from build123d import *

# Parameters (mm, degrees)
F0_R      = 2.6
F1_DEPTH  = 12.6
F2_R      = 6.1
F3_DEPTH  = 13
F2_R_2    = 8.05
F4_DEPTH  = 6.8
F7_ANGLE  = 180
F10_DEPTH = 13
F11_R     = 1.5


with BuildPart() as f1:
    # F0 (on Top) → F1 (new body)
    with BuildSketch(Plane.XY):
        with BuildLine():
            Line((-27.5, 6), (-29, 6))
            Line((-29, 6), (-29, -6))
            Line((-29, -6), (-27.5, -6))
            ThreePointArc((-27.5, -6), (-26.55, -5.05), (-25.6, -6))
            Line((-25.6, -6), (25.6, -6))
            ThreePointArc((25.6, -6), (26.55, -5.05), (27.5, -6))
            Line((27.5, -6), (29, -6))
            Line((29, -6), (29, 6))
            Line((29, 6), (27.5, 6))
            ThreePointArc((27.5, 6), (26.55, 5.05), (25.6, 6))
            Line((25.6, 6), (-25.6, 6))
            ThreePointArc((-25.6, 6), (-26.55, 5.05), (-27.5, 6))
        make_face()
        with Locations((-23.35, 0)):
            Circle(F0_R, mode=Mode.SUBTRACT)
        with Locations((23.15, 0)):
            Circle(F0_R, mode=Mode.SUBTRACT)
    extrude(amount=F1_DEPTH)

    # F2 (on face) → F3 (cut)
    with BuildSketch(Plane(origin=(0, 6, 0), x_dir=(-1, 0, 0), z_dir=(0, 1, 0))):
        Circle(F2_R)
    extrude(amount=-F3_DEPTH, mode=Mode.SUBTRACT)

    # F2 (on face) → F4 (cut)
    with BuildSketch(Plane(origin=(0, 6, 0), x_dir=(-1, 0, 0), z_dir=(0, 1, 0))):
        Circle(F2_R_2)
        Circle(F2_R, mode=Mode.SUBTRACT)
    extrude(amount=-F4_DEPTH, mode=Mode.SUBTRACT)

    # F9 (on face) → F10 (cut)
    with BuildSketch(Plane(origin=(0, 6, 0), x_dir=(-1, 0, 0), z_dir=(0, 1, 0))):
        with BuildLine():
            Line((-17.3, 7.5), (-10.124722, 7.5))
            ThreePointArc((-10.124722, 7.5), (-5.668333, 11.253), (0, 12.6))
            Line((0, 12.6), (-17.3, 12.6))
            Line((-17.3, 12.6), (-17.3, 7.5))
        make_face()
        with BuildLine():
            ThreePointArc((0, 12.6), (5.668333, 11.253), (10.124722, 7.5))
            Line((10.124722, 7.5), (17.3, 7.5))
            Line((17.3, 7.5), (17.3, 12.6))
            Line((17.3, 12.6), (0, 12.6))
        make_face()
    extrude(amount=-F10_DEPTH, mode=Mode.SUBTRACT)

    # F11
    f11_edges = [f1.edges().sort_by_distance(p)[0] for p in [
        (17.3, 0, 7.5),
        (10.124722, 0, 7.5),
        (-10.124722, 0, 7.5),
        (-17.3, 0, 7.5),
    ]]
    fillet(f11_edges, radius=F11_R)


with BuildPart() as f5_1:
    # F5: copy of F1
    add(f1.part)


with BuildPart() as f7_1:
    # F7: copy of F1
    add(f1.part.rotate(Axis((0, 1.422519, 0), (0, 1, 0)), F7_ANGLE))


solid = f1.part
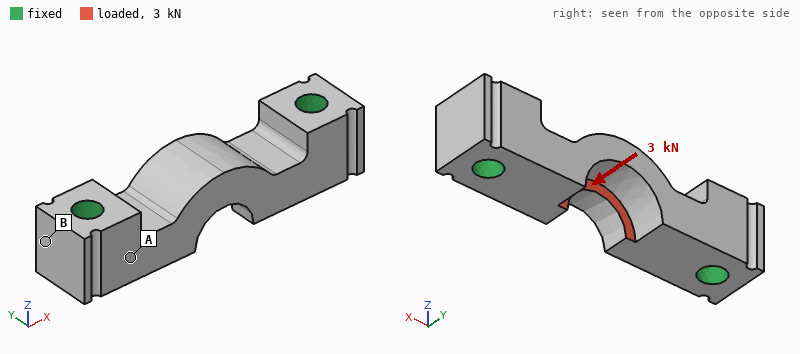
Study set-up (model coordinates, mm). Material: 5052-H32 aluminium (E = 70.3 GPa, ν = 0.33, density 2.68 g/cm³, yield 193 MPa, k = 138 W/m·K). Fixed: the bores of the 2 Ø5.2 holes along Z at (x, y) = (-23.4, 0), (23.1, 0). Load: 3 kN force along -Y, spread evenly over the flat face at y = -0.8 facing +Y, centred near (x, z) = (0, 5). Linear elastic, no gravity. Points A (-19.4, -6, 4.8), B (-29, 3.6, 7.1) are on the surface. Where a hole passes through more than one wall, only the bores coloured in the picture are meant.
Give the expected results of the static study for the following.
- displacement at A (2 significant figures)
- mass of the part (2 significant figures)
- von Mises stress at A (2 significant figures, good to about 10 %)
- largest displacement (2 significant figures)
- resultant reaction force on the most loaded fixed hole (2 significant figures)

7.5 µm
16 g
64 MPa
46 µm
1.5 kN
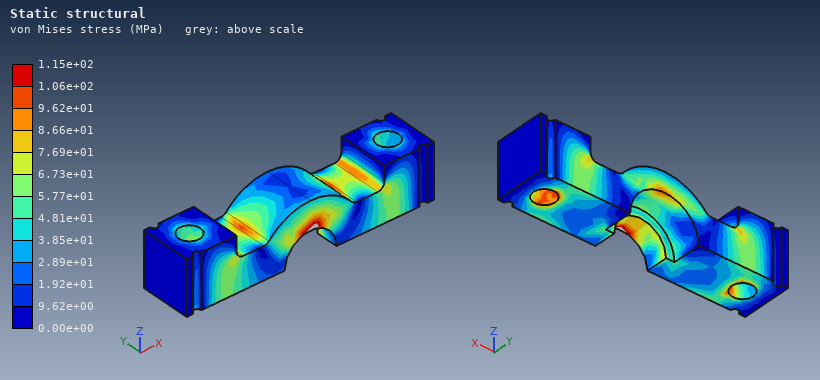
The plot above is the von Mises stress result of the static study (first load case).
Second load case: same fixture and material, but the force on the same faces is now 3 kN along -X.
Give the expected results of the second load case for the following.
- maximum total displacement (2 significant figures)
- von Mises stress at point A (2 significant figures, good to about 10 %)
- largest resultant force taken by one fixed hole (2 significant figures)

9.8 µm
14 MPa
1.5 kN
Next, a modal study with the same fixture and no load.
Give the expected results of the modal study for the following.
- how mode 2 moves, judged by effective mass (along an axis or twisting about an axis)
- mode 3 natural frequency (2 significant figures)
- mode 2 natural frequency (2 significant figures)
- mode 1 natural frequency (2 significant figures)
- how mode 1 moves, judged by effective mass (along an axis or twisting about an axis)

along Z
35 kHz
23 kHz
18 kHz
along Y
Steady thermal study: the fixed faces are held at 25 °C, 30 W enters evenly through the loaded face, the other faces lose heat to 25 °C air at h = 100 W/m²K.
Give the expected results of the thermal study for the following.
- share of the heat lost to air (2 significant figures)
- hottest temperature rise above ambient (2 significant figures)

6.9 %
28 K
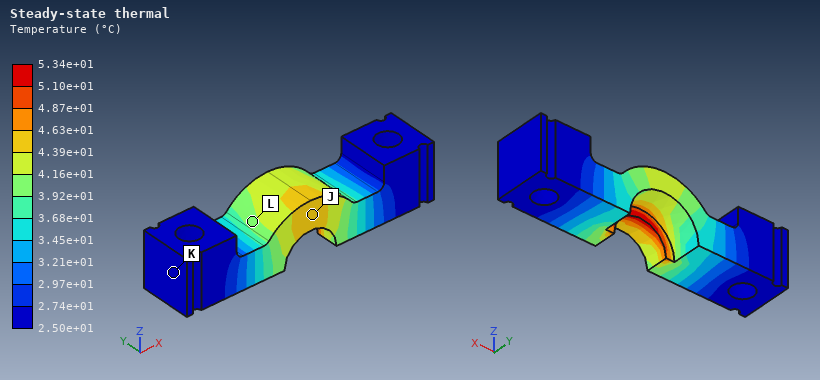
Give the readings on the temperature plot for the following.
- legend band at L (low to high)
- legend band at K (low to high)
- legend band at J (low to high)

3.92e+01 to 4.16e+01 °C
2.50e+01 to 2.74e+01 °C
4.39e+01 to 4.63e+01 °C
